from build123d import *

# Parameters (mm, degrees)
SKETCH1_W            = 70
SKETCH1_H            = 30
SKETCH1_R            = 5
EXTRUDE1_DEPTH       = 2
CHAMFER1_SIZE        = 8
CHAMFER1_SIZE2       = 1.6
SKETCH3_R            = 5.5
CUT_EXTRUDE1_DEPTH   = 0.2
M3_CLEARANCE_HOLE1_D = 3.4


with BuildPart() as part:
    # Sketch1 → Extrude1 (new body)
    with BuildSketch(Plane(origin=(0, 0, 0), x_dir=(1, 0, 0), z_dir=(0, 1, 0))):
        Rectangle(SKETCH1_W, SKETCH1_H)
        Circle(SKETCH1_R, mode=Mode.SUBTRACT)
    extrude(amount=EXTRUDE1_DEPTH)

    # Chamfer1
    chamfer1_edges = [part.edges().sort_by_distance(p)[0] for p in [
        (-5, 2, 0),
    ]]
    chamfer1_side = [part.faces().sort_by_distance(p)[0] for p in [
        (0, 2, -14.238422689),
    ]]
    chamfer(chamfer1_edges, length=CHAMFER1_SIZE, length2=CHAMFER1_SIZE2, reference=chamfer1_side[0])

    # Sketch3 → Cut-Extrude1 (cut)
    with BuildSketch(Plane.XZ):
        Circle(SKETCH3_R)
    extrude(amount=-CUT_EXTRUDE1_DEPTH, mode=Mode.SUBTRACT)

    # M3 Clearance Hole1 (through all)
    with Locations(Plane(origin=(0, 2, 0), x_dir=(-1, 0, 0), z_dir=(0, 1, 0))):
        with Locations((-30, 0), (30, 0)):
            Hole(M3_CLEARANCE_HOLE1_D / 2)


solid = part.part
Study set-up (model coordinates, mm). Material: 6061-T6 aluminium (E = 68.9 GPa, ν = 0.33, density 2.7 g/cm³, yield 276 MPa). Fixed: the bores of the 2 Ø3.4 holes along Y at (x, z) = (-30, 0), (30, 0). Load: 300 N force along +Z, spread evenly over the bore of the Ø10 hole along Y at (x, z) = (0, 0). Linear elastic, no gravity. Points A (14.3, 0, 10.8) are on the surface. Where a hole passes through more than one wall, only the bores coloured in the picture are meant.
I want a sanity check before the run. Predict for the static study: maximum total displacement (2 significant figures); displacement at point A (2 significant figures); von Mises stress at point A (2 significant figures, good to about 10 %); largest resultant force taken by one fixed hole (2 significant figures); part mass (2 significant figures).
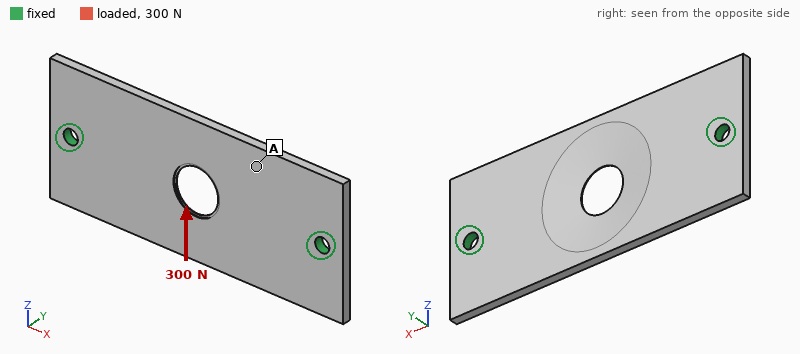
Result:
22 µm
12 µm
8.5 MPa
150 N
10.0 g
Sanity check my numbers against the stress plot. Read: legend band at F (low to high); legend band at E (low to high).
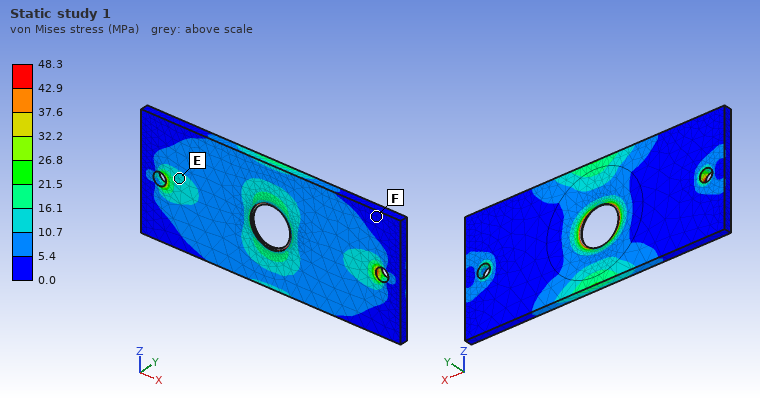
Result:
0.0 to 5.4 MPa
10.7 to 16.1 MPa
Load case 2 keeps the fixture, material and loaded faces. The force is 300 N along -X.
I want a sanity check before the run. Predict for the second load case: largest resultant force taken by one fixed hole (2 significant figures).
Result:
150 N
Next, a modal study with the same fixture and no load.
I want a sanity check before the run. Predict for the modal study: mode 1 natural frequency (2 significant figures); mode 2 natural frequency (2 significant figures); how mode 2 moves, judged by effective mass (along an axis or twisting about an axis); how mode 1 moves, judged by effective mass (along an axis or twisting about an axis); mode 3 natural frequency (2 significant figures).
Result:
2700 Hz
3200 Hz
twisting about X
along Y
5900 Hz
